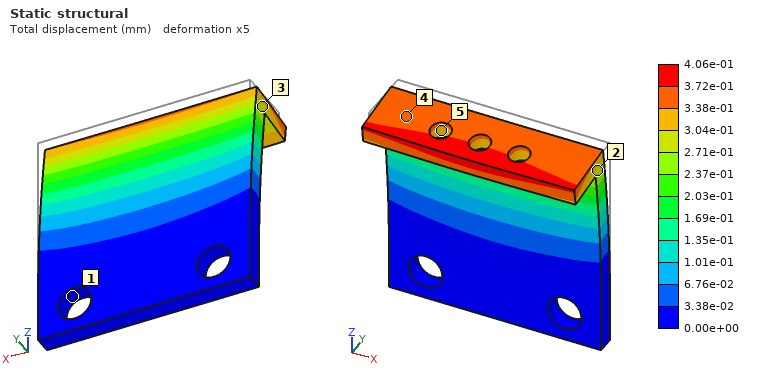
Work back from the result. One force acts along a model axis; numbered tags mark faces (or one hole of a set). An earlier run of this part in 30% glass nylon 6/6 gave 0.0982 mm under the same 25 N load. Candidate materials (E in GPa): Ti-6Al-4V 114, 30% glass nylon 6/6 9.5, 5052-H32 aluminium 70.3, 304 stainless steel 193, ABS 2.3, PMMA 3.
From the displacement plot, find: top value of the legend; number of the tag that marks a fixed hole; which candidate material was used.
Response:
4.06e-01 mm
1
ABS
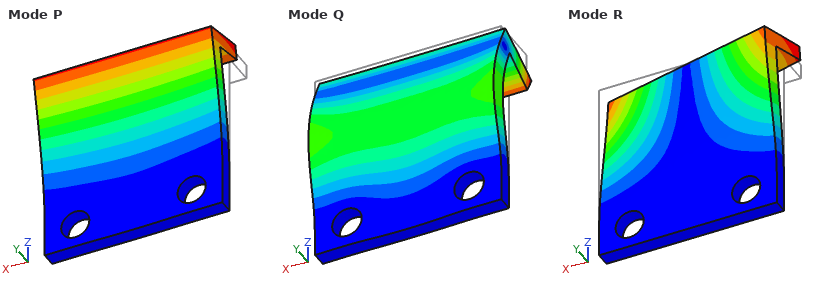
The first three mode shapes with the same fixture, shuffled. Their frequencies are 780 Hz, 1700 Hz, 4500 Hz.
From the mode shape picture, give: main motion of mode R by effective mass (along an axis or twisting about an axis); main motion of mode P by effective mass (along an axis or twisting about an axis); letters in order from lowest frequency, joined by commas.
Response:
twisting about Z
along Y
P, R, Q
